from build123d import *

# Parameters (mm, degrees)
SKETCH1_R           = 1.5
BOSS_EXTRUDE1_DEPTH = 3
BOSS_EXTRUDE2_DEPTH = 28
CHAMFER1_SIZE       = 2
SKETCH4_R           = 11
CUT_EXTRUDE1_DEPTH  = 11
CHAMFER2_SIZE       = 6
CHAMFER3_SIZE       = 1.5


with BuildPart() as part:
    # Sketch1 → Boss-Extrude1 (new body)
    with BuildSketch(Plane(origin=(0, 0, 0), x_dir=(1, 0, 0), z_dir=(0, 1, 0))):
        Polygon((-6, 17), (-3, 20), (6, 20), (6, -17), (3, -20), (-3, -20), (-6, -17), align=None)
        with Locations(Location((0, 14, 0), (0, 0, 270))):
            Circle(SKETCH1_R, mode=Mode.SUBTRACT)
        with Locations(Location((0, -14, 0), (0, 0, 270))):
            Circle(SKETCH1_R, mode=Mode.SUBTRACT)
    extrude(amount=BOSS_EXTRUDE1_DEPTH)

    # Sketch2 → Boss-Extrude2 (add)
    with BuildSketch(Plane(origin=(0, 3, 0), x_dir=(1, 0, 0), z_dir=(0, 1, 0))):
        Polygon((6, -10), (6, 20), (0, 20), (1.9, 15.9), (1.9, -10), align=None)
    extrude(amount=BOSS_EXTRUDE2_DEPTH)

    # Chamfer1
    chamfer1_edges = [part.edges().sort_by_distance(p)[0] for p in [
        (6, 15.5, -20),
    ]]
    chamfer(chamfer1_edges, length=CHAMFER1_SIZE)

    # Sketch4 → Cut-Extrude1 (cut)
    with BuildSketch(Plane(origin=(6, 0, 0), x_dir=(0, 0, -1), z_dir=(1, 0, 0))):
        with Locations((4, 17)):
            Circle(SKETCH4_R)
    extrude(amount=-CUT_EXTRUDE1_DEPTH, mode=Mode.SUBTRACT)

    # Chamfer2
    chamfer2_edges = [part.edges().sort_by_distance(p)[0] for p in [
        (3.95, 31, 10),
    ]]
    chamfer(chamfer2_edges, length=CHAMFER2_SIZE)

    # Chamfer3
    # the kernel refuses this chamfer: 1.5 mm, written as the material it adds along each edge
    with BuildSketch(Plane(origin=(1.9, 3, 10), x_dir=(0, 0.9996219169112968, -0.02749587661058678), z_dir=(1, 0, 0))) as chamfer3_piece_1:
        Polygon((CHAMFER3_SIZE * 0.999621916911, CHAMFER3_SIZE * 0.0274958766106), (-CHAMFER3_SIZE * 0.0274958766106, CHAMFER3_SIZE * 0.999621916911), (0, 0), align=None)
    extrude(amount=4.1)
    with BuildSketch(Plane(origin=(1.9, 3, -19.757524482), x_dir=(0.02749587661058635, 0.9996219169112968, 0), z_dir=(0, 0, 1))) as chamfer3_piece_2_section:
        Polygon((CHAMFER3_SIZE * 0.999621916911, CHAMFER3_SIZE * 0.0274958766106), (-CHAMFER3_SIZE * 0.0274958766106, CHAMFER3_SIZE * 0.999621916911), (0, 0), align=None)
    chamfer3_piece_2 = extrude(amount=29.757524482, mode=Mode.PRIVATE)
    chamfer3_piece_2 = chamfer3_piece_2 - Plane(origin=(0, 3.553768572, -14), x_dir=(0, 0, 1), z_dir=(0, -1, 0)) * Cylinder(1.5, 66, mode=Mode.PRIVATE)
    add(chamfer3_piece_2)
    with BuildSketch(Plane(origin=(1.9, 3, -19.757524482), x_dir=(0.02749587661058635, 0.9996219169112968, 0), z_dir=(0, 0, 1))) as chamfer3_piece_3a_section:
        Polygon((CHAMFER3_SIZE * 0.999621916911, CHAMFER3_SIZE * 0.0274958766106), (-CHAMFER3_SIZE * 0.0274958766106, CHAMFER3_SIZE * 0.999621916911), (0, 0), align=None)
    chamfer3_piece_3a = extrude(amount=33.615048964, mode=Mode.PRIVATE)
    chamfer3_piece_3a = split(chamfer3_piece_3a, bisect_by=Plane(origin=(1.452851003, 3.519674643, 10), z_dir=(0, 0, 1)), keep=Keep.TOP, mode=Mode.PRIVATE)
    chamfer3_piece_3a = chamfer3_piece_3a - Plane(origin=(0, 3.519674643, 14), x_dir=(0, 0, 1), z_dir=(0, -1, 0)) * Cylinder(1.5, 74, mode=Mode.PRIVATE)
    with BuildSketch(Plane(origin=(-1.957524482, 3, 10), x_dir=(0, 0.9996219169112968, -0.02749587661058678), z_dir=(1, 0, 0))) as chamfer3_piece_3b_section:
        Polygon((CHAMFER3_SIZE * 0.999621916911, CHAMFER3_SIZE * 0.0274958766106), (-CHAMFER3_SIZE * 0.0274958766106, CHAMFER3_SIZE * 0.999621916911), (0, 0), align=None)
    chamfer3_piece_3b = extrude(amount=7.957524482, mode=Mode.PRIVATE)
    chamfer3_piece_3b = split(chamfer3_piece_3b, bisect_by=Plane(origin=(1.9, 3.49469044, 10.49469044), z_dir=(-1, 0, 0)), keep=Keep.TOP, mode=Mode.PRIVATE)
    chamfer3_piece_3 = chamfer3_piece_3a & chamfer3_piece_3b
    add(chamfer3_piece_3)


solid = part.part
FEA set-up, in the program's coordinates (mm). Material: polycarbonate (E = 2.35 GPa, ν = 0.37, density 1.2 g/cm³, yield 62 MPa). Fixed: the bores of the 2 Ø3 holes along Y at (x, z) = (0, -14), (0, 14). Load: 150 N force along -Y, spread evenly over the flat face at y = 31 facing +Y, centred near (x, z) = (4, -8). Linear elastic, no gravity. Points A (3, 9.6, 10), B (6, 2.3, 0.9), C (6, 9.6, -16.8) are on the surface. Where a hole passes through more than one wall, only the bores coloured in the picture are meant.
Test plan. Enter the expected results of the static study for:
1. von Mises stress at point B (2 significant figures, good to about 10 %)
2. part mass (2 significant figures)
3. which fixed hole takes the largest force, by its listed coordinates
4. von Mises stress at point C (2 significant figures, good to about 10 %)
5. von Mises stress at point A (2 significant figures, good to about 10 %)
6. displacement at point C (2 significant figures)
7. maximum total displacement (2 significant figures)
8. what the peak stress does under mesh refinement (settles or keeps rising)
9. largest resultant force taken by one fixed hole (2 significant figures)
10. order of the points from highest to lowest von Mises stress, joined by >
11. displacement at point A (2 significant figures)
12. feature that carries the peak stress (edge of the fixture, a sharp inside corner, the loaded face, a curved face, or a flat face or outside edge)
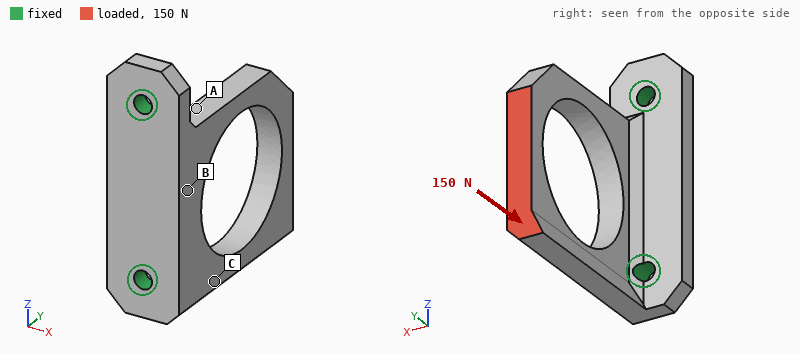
2.3 MPa
3.9 g
(0, -14)
5.7 MPa
9.4 MPa
0.096 mm
0.33 mm
keeps rising
110 N
A > C > B
0.080 mm
edge of the fixture
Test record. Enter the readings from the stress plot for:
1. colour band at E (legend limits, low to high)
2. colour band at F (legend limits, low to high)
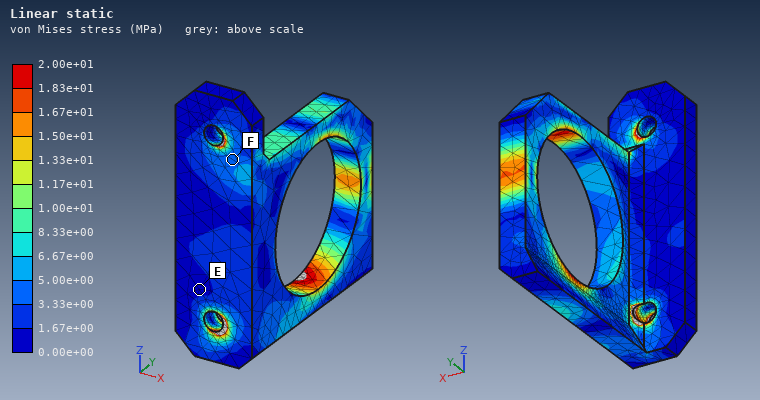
0.00e+00 to 1.67e+00 MPa
3.33e+00 to 5.00e+00 MPa
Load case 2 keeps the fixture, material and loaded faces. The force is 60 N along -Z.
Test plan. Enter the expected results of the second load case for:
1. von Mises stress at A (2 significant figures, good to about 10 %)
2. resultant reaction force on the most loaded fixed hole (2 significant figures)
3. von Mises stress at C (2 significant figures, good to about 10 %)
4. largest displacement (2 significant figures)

15 MPa
66 N
4.8 MPa
0.50 mm
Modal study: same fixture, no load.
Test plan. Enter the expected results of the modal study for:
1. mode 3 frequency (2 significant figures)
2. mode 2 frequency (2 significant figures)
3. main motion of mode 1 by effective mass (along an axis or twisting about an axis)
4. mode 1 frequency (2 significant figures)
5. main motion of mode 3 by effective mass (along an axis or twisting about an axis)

2200 Hz
1800 Hz
along X
860 Hz
along Z
